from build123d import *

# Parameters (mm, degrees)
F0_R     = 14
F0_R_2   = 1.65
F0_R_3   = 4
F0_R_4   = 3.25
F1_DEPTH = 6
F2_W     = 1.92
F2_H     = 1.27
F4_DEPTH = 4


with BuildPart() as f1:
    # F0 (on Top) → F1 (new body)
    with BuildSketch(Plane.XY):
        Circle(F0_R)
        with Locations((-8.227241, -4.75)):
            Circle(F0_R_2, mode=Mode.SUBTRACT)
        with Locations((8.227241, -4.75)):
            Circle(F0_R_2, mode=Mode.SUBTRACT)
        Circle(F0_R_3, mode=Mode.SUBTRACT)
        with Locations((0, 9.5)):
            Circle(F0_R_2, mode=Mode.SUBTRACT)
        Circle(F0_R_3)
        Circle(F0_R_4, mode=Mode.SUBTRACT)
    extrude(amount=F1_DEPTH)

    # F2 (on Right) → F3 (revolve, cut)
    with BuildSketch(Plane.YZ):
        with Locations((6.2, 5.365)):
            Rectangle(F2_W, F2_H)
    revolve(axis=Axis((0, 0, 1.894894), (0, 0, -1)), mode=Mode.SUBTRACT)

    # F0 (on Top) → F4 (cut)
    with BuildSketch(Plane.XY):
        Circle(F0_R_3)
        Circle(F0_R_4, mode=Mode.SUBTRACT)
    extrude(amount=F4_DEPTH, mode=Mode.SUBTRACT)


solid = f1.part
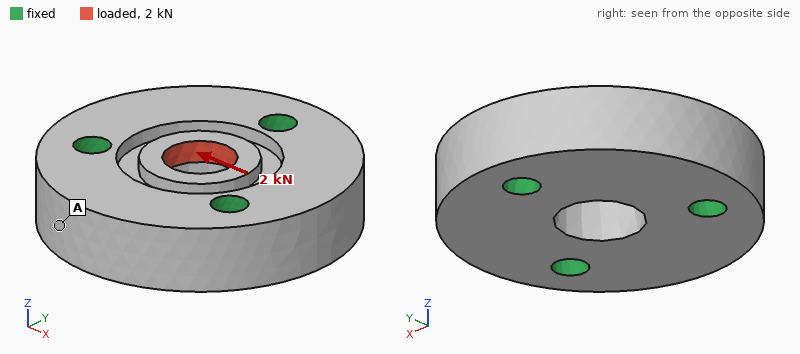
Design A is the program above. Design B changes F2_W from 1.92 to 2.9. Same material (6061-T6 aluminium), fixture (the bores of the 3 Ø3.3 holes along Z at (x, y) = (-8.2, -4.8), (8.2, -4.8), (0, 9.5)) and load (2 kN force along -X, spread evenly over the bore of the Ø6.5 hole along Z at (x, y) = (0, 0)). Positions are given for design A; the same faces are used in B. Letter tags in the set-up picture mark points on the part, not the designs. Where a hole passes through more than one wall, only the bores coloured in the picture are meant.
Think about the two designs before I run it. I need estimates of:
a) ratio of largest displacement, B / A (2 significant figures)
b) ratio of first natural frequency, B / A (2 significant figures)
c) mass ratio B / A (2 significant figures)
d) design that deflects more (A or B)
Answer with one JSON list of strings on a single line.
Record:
["1.3", "0.99", "0.98", "B"]
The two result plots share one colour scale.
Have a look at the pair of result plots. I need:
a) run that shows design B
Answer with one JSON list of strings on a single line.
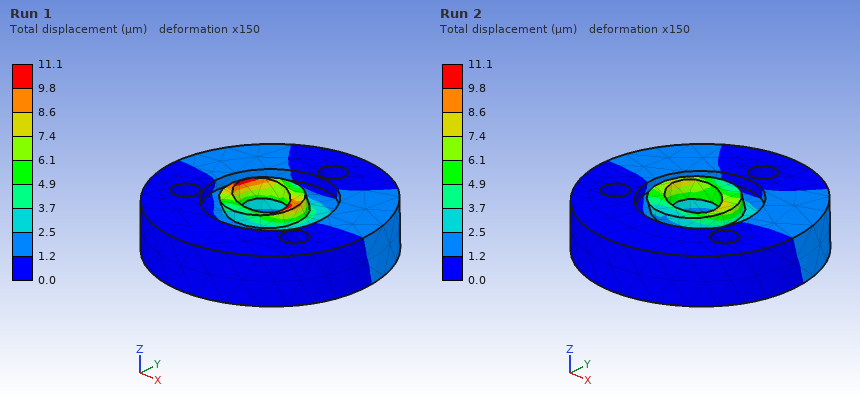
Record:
["Run 1"]
